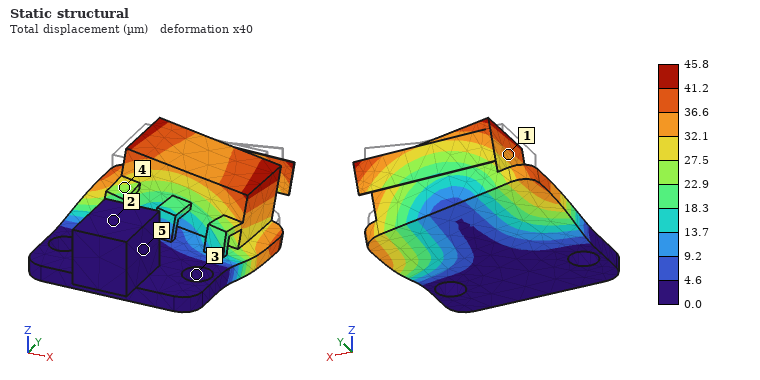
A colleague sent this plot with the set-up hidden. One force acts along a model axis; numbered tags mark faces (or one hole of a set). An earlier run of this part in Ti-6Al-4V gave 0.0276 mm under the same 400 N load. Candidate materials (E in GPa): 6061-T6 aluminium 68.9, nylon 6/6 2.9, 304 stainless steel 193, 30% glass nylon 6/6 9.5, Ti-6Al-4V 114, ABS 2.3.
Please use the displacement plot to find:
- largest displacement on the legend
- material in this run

45.8 µm
6061-T6 aluminium
